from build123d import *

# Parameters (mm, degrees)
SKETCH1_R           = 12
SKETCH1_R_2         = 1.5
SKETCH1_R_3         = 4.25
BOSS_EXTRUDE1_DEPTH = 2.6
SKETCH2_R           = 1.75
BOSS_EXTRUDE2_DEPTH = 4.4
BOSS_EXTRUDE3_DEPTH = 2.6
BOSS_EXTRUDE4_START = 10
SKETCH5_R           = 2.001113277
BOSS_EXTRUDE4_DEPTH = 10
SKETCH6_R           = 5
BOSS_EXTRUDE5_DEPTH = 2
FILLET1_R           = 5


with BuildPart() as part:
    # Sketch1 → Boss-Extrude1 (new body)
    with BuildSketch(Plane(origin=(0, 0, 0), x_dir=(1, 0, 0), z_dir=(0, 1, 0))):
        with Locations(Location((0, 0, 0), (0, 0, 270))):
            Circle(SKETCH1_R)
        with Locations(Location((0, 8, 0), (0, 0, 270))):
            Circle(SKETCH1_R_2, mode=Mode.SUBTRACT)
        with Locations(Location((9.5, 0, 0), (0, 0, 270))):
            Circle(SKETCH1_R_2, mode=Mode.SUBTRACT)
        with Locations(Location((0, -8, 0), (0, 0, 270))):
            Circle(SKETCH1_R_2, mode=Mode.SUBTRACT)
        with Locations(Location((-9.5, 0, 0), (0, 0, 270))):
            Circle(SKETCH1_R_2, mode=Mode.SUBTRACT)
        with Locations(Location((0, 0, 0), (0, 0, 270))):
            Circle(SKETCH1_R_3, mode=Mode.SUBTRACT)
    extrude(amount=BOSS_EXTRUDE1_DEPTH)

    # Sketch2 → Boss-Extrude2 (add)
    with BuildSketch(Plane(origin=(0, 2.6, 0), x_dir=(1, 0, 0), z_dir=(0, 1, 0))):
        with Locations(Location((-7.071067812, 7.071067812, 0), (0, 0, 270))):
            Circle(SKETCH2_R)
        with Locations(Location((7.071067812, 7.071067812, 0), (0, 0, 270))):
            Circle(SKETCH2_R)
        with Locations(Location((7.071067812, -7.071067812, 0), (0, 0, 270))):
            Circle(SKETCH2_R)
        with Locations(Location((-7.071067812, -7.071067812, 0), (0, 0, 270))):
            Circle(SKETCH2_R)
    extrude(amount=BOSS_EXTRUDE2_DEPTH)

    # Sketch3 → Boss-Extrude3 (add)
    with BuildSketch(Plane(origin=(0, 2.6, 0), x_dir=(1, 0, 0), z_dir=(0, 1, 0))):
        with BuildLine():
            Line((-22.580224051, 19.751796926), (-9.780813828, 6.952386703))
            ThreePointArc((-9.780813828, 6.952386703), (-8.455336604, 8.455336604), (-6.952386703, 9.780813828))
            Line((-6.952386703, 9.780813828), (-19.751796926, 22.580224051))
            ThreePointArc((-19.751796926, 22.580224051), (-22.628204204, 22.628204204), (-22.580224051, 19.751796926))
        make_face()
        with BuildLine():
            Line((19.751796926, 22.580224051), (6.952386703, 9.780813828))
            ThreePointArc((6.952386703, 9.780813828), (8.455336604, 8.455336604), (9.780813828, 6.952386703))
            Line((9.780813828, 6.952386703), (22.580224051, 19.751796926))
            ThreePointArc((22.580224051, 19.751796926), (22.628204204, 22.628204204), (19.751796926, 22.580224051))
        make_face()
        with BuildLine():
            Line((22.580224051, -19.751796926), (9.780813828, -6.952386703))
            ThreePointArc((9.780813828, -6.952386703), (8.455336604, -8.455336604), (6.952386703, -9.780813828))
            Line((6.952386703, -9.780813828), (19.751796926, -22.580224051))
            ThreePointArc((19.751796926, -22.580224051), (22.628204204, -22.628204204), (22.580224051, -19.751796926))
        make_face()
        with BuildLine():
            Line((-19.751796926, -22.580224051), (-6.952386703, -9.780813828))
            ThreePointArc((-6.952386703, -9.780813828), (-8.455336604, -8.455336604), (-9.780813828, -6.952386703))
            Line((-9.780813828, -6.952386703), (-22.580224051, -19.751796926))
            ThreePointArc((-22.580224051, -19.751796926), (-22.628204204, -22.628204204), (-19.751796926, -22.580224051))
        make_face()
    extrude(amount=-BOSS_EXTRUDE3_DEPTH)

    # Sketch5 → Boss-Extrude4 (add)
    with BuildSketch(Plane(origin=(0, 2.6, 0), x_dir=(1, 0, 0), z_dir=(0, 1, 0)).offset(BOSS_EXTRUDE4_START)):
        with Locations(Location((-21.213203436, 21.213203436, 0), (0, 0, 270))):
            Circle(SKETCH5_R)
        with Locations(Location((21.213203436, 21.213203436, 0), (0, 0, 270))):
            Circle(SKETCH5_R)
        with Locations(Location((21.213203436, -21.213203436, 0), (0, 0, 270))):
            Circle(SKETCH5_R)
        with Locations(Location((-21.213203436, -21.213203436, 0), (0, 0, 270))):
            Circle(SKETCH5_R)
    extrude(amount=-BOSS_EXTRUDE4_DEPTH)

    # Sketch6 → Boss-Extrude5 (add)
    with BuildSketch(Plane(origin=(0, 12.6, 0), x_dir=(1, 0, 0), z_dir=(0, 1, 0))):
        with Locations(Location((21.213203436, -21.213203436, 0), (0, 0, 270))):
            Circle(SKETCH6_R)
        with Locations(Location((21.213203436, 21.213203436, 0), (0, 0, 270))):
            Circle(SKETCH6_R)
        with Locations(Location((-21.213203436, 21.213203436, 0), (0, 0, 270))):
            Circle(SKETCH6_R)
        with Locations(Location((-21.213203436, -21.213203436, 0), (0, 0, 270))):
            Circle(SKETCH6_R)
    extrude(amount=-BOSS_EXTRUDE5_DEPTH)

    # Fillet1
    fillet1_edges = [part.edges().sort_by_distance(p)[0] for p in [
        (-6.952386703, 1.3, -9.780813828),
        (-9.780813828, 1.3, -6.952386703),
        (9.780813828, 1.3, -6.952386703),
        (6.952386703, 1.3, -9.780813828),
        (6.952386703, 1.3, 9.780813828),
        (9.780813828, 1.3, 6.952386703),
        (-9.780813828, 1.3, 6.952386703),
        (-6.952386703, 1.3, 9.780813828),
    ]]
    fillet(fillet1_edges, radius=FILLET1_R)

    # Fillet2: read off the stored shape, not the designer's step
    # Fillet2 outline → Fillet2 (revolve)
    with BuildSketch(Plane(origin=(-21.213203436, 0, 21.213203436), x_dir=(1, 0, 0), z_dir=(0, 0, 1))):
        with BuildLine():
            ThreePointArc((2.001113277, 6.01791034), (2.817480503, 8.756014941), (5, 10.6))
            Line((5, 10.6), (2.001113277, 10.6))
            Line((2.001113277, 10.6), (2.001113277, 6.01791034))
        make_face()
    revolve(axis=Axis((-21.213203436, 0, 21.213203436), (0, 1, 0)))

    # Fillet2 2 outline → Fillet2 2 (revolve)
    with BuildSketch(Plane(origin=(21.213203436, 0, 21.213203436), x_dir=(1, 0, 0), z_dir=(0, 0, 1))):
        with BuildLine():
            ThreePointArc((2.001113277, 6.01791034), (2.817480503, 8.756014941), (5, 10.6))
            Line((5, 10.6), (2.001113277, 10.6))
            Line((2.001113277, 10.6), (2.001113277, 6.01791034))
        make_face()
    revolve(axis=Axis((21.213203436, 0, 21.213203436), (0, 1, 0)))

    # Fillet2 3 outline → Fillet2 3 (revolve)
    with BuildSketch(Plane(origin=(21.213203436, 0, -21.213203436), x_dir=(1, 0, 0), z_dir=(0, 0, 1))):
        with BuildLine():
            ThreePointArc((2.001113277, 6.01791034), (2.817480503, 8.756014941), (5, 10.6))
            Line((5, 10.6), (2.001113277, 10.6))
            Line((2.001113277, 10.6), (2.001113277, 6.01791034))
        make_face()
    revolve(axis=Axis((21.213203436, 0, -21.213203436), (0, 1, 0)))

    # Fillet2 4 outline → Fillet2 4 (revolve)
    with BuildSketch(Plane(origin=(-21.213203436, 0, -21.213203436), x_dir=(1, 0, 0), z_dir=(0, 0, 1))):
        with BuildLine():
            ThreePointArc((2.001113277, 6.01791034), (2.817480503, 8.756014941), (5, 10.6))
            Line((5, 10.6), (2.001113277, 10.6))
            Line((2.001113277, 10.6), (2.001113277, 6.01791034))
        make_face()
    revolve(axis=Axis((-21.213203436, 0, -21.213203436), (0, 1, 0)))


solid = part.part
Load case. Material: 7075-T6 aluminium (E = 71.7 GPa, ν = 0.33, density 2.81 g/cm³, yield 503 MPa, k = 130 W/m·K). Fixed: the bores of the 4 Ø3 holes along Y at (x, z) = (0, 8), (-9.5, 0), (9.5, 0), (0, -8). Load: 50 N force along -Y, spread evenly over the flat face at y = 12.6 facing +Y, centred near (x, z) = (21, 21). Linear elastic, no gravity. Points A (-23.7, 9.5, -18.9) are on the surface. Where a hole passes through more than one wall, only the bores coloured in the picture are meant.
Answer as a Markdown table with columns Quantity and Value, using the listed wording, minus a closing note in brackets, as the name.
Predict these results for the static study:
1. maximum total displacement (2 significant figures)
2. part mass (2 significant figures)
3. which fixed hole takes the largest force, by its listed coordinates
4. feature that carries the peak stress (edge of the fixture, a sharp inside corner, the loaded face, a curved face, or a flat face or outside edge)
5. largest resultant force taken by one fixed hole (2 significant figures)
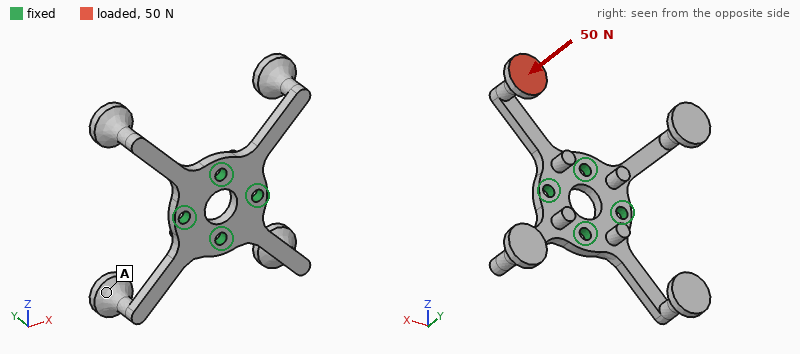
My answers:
| Quantity | Value |
|---|---|
| maximum total displacement | 0.53 mm |
| part mass | 9.2 g |
| which fixed hole takes the largest force, by its listed coordinates | (9.5, 0) |
| feature that carries the peak stress | a curved face |
| largest resultant force taken by one fixed hole | 38 N |
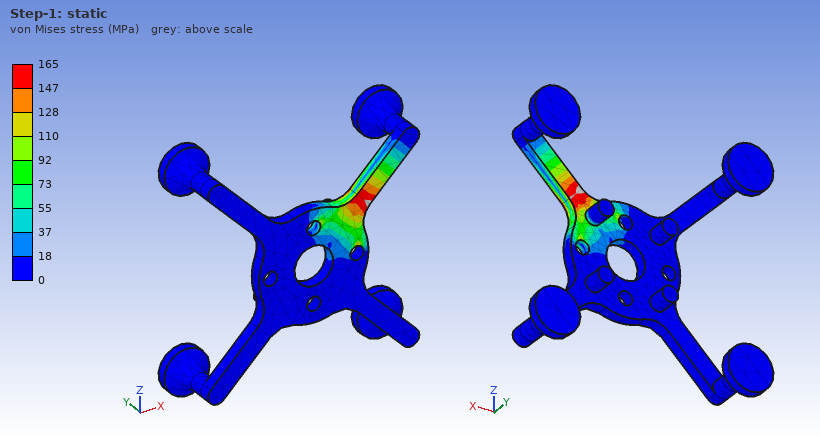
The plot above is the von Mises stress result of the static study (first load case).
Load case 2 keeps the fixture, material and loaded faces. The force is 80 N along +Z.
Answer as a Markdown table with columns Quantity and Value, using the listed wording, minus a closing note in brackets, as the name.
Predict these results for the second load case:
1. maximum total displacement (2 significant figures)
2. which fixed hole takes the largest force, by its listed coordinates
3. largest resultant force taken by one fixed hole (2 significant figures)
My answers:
| Quantity | Value |
|---|---|
| maximum total displacement | 0.78 mm |
| which fixed hole takes the largest force, by its listed coordinates | (9.5, 0) |
| largest resultant force taken by one fixed hole | 150 N |
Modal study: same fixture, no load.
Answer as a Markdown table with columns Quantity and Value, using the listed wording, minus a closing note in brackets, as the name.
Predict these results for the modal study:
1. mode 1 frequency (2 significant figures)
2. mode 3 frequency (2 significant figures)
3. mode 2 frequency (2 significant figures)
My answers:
| Quantity | Value |
|---|---|
| mode 1 frequency | 1600 Hz |
| mode 3 frequency | 1600 Hz |
| mode 2 frequency | 1600 Hz |
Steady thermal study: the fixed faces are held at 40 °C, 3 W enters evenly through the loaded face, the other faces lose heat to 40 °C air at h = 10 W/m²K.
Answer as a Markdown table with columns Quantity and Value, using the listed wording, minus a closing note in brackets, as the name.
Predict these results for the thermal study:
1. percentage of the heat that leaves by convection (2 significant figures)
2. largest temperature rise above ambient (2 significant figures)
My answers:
| Quantity | Value |
|---|---|
| percentage of the heat that leaves by convection | 6.0 % |
| largest temperature rise above ambient | 54 K |
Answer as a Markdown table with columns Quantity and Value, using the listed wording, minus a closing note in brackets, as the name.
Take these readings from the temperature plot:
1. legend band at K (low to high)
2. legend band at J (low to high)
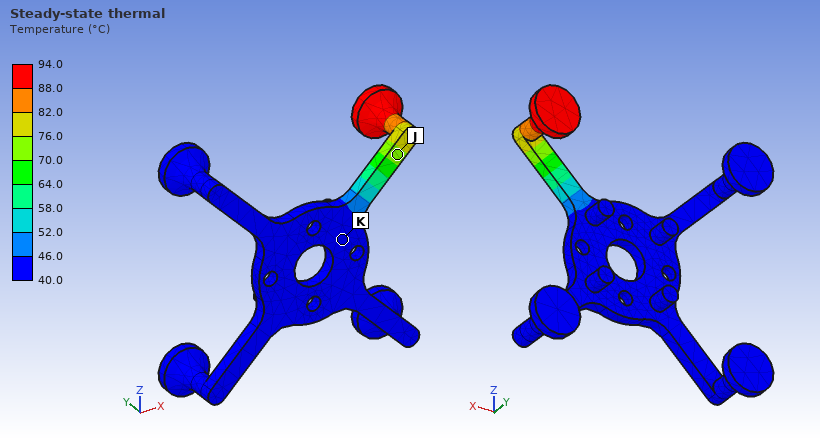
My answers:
| Quantity | Value |
|---|---|
| legend band at K | 40.0 to 46.0 °C |
| legend band at J | 70.0 to 76.0 °C |
